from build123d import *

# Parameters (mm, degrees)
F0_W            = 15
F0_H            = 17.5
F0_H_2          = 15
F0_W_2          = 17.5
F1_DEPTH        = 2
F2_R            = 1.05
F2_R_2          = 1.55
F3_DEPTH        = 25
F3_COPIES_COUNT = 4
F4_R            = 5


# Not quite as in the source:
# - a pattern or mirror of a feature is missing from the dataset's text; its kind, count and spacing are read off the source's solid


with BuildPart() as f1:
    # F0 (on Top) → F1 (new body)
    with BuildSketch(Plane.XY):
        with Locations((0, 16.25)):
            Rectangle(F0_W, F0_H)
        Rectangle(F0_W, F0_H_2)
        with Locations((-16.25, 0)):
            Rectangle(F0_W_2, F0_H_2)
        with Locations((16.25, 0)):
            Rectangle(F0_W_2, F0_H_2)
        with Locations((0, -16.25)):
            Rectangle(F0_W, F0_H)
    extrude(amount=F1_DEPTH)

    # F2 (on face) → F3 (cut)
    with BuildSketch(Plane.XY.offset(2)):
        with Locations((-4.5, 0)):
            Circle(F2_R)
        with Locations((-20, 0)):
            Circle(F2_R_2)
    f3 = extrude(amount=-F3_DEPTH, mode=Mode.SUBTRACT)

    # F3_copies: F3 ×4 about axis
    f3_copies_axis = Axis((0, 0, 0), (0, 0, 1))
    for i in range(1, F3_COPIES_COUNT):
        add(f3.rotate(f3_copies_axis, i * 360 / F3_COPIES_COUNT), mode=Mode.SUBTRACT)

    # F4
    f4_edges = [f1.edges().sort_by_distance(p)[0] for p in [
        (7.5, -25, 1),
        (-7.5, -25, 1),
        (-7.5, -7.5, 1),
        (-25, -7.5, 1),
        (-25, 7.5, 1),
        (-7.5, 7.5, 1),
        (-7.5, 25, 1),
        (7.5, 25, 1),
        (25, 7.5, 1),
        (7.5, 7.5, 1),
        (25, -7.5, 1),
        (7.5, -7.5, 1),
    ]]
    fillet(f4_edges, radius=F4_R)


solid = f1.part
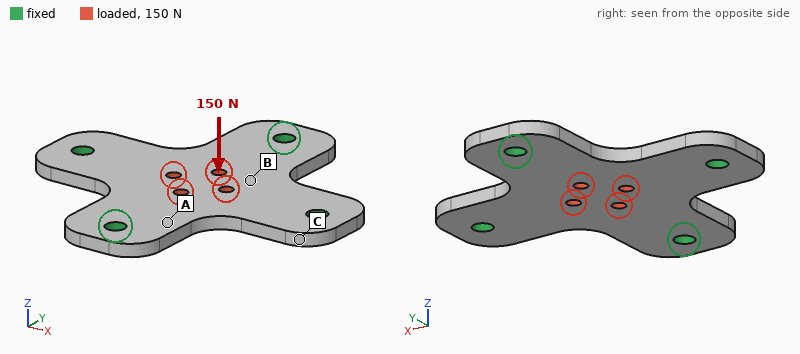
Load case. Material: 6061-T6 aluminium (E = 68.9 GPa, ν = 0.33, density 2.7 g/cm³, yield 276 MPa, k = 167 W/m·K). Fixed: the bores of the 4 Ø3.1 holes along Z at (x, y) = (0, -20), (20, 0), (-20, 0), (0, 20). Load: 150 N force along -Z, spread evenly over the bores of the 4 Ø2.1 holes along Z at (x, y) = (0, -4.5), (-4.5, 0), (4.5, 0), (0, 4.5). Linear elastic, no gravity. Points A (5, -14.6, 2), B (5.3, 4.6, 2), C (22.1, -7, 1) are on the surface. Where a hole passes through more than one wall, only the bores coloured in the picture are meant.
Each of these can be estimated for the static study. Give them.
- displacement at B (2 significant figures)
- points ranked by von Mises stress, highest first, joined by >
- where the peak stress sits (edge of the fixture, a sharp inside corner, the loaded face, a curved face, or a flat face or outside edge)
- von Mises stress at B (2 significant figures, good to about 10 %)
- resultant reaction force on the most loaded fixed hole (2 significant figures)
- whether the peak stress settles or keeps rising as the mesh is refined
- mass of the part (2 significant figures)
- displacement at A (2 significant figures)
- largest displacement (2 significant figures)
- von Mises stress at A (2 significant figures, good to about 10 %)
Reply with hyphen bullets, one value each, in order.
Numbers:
- 21 µm
- B > A > C
- edge of the fixture
- 19 MPa
- 38 N
- keeps rising
- 6.5 g
- 5.1 µm
- 29 µm
- 12 MPa
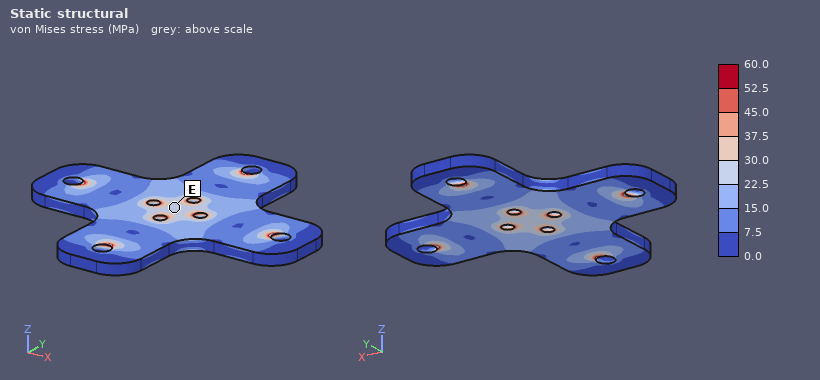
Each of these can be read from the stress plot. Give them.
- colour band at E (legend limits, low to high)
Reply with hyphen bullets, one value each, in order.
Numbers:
- 22.5 to 30.0 MPa
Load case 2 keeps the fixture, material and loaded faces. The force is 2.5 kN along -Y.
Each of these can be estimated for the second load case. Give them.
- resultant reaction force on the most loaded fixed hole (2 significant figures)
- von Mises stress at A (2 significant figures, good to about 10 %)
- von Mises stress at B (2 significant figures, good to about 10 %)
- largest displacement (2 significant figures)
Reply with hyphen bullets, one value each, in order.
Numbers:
- 1.1 kN
- 30 MPa
- 32 MPa
- 14 µm
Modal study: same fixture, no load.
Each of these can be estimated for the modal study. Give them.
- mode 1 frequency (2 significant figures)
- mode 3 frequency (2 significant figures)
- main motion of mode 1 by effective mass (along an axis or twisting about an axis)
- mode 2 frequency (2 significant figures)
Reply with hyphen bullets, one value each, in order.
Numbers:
- 9600 Hz
- 18 kHz
- along Z
- 18 kHz
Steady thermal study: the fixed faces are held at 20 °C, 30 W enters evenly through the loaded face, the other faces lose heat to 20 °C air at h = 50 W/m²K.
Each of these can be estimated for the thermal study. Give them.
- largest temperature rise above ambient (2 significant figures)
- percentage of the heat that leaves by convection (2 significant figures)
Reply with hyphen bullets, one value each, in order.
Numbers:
- 31 K
- 4.8 %
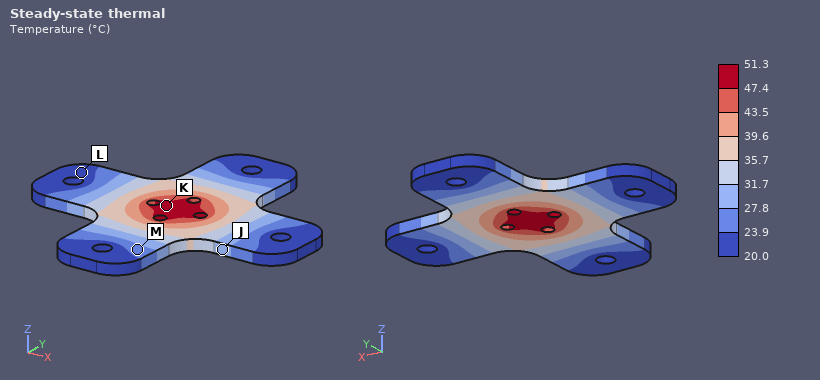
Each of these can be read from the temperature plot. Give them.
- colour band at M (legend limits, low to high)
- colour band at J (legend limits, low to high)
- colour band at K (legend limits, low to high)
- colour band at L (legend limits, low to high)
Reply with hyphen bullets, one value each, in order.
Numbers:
- 23.9 to 27.8 °C
- 27.8 to 31.7 °C
- 47.4 to 51.3 °C
- 20.0 to 23.9 °C
